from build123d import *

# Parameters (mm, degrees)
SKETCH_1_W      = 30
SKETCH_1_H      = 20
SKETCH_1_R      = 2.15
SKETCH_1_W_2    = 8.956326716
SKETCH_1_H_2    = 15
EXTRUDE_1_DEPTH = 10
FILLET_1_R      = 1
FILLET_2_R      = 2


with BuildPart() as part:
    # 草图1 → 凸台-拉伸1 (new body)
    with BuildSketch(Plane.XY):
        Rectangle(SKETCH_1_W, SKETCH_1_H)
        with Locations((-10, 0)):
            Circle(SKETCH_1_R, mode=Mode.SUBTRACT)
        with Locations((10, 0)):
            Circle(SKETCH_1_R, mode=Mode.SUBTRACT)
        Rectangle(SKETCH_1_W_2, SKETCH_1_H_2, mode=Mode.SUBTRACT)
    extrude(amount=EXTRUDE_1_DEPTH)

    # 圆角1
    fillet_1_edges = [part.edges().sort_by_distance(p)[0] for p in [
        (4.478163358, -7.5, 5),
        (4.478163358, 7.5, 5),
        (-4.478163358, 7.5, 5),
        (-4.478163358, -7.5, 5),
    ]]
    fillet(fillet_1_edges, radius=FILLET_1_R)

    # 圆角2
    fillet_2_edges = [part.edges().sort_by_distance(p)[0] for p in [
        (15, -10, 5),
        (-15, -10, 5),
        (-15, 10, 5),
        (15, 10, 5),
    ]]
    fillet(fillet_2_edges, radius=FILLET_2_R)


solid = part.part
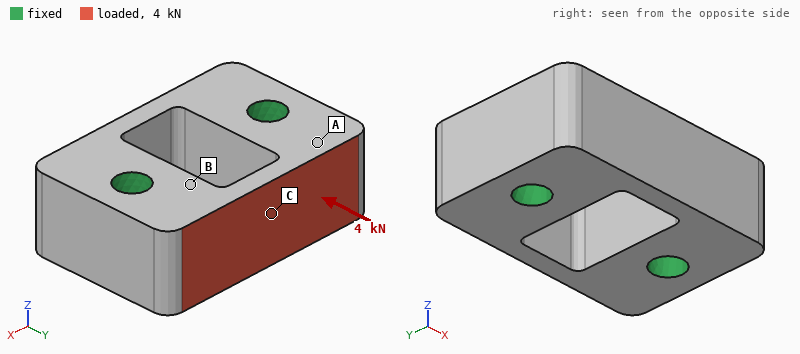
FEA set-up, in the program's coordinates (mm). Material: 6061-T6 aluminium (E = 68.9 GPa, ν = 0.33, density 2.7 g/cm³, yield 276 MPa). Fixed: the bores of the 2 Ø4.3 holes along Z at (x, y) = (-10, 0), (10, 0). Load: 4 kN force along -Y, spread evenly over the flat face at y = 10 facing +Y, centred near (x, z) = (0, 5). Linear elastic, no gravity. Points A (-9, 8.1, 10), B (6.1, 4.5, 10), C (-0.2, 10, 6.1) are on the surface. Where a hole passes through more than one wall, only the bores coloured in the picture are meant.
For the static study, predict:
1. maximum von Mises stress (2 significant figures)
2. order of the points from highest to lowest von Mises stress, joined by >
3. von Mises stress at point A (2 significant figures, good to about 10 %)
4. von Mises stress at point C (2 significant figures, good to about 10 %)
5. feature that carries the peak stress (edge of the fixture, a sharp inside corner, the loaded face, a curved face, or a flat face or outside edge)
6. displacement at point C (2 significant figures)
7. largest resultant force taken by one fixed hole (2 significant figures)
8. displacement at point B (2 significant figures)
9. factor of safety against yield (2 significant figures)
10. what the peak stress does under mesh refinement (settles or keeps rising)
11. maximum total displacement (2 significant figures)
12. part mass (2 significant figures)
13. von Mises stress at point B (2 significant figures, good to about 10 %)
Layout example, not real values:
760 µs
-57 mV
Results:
150 MPa
C > B > A
14 MPa
77 MPa
a curved face
12 µm
2.1 kN
2.4 µm
1.9
settles
14 µm
12 g
35 MPa
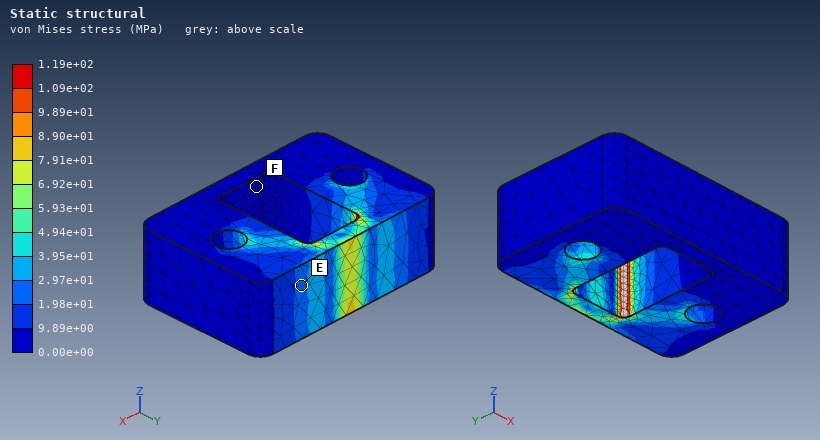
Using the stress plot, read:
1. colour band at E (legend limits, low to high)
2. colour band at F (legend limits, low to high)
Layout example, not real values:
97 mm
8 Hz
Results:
1.98e+01 to 2.97e+01 MPa
0.00e+00 to 9.89e+00 MPa
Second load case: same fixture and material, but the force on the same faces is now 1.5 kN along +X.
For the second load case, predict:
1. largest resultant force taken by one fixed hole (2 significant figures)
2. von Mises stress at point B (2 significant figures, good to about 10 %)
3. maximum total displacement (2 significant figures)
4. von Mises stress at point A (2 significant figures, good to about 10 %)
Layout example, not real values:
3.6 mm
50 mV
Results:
780 N
15 MPa
6.9 µm
13 MPa
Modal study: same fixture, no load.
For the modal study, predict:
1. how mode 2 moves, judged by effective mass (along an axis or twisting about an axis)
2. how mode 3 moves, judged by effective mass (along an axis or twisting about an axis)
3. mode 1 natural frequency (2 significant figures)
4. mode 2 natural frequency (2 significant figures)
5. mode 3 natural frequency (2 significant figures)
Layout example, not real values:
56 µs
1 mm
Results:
twisting about X
along Z
41 kHz
49 kHz
52 kHz
